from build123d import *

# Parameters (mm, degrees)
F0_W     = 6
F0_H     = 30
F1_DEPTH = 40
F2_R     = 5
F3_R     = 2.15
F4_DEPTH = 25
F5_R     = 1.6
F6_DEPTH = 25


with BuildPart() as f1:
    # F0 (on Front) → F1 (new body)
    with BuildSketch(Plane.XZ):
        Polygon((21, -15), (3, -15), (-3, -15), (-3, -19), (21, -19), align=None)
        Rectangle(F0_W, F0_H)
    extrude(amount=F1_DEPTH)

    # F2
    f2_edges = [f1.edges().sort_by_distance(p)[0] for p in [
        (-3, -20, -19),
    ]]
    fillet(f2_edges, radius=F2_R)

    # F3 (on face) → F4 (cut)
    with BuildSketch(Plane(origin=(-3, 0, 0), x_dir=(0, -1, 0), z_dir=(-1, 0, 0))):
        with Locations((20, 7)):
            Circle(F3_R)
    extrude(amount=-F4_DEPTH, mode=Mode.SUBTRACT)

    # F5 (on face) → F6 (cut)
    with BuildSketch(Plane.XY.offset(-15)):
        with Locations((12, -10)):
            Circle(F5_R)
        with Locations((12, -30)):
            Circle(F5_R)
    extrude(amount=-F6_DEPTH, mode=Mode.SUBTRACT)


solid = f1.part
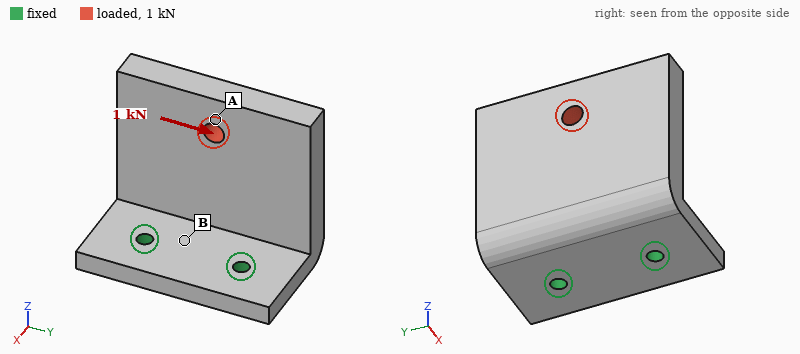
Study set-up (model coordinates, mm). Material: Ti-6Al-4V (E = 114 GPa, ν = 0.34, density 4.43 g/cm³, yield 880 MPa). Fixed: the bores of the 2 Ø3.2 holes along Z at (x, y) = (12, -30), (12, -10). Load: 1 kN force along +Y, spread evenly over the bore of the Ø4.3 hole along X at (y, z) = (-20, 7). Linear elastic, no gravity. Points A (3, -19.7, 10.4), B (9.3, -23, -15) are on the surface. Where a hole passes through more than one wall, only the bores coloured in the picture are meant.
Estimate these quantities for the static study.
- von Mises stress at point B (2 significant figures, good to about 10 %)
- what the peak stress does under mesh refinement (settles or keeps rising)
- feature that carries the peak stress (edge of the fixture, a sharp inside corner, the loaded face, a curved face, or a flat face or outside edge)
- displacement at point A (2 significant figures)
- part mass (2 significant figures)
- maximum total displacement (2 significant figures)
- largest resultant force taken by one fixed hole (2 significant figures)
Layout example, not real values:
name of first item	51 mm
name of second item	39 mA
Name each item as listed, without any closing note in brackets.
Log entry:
von Mises stress at point B	50 MPa
what the peak stress does under mesh refinement	keeps rising
feature that carries the peak stress	edge of the fixture
displacement at point A	61 µm
part mass	47 g
maximum total displacement	82 µm
largest resultant force taken by one fixed hole	1.2 kN
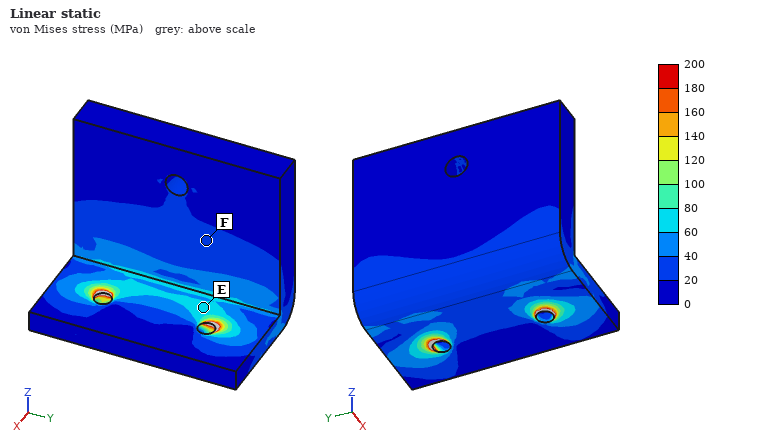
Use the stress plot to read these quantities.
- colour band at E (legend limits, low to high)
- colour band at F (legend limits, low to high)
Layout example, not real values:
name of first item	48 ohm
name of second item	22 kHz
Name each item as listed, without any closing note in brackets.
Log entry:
colour band at E	60 to 80 MPa
colour band at F	20 to 40 MPa
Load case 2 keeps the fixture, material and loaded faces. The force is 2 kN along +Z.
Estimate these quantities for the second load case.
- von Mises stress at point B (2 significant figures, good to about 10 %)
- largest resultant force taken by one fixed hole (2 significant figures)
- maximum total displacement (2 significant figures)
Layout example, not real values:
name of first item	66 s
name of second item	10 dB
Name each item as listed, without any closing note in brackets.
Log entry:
von Mises stress at point B	100 MPa
largest resultant force taken by one fixed hole	1.0 kN
maximum total displacement	0.23 mm
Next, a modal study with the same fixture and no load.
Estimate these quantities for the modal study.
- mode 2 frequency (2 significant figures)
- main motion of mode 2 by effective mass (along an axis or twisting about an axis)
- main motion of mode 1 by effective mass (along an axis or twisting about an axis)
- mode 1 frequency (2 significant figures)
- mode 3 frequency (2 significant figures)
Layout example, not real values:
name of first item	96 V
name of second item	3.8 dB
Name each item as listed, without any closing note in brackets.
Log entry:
mode 2 frequency	4200 Hz
main motion of mode 2 by effective mass	along Y
main motion of mode 1 by effective mass	along X
mode 1 frequency	1900 Hz
mode 3 frequency	7700 Hz
